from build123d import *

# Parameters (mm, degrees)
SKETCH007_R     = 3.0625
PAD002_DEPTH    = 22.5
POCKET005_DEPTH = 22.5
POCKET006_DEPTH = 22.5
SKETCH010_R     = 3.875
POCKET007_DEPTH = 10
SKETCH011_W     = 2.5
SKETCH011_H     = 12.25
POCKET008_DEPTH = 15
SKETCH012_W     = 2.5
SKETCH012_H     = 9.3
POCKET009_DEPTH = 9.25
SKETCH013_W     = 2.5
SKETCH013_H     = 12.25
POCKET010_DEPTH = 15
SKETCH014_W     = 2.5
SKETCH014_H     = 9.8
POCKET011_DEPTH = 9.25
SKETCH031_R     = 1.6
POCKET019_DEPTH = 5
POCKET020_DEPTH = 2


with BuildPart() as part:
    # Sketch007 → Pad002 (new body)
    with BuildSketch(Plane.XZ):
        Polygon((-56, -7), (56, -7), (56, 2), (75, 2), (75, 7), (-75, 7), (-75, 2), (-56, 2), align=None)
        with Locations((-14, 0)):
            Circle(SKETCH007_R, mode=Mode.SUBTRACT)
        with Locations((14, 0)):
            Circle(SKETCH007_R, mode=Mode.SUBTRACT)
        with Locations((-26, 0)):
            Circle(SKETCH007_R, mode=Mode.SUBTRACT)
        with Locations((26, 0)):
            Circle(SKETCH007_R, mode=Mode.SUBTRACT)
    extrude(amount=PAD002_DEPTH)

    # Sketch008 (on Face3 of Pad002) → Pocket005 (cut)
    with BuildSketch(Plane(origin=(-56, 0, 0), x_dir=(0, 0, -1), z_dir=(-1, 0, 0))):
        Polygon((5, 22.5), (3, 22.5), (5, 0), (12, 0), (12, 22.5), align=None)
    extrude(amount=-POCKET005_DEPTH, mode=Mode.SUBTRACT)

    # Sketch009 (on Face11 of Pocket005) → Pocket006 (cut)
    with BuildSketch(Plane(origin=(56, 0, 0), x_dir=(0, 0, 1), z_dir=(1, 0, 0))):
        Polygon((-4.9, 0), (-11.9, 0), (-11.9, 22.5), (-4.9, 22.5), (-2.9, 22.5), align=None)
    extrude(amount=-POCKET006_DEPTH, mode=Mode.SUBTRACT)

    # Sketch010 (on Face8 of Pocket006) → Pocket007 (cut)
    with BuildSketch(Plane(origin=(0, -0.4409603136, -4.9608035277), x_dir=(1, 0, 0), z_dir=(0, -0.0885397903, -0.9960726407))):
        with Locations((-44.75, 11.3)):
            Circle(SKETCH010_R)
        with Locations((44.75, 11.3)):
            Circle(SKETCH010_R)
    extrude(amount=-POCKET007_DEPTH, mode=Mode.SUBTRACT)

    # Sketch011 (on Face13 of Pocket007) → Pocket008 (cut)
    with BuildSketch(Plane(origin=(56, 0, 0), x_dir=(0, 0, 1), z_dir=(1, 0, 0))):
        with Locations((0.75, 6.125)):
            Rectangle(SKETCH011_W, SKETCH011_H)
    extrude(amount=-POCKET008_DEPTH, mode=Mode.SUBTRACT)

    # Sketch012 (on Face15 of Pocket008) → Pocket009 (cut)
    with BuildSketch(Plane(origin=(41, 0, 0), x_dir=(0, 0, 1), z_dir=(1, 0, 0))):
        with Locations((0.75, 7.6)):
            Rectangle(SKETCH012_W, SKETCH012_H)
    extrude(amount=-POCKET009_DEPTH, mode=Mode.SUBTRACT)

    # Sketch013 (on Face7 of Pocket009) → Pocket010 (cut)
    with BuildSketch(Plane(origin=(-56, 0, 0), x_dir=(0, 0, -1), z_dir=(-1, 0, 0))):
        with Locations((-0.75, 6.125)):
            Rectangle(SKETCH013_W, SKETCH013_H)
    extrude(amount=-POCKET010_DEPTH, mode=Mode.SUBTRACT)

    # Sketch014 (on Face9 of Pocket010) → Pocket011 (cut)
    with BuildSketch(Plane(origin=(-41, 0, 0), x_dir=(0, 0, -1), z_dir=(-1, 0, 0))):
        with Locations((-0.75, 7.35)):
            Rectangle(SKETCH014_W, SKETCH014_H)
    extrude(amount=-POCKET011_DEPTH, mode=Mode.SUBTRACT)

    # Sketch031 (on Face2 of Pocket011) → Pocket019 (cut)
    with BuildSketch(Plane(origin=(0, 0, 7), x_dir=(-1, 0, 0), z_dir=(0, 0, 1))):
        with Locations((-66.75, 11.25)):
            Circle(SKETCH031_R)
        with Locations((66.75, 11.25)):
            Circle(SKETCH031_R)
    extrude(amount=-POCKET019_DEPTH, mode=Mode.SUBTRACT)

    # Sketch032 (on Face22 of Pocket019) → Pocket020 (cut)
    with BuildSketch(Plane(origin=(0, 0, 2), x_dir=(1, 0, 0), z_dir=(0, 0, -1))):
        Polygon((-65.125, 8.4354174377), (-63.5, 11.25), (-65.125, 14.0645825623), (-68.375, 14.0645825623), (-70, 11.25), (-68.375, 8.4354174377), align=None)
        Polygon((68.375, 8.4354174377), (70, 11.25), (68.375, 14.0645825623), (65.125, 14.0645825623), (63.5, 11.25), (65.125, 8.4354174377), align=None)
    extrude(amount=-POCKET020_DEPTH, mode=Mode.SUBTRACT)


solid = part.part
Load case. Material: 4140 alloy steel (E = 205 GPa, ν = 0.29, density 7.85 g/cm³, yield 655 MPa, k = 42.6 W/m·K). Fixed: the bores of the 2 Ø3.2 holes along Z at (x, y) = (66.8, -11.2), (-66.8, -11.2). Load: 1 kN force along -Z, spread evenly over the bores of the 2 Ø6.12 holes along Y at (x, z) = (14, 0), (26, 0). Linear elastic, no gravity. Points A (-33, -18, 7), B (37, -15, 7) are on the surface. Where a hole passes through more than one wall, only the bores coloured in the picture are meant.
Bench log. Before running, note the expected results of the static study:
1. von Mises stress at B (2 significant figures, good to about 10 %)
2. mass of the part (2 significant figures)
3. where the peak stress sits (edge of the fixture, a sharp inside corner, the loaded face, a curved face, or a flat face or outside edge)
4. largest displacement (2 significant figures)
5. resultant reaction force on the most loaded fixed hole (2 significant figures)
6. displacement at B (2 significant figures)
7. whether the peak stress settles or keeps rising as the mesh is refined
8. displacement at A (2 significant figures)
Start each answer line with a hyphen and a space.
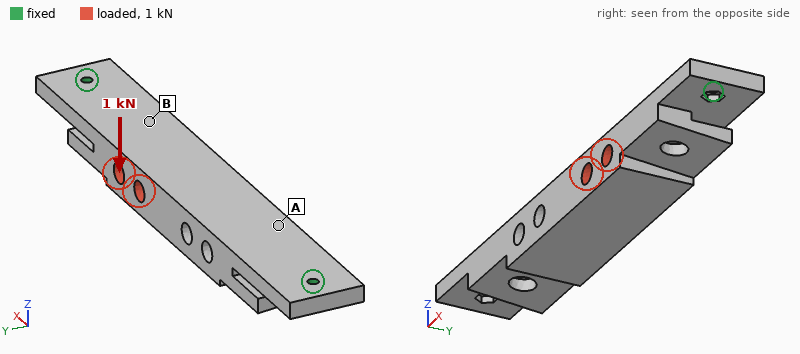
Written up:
- 28 MPa
- 250 g
- edge of the fixture
- 41 µm
- 1.4 kN
- 30 µm
- keeps rising
- 21 µm
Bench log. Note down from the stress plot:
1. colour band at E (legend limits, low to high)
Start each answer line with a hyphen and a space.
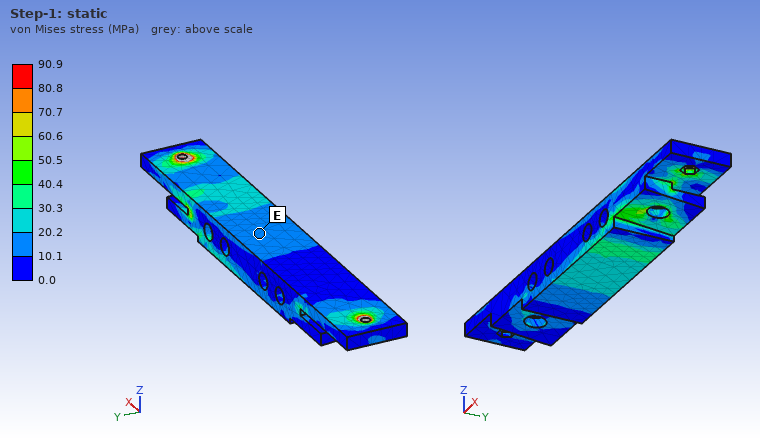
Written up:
- 10.1 to 20.2 MPa
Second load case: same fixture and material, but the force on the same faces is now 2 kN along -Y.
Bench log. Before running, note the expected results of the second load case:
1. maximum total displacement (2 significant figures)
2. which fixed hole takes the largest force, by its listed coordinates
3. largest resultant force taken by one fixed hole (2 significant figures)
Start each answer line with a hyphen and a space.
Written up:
- 73 µm
- (66.8, -11.2)
- 1.3 kN
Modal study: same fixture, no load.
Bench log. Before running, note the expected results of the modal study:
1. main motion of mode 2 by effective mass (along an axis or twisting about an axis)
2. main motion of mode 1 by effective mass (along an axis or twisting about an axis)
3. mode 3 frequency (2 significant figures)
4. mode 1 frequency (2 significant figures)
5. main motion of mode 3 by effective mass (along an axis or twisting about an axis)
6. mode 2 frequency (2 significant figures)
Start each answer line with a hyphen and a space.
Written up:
- along Y
- along Z
- 3700 Hz
- 2000 Hz
- along Y
- 2200 Hz
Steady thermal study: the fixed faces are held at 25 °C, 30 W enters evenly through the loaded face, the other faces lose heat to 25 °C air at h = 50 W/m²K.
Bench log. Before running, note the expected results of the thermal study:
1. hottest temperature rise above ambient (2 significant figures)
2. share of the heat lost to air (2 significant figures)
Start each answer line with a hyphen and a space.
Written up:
- 66 K
- 68 %
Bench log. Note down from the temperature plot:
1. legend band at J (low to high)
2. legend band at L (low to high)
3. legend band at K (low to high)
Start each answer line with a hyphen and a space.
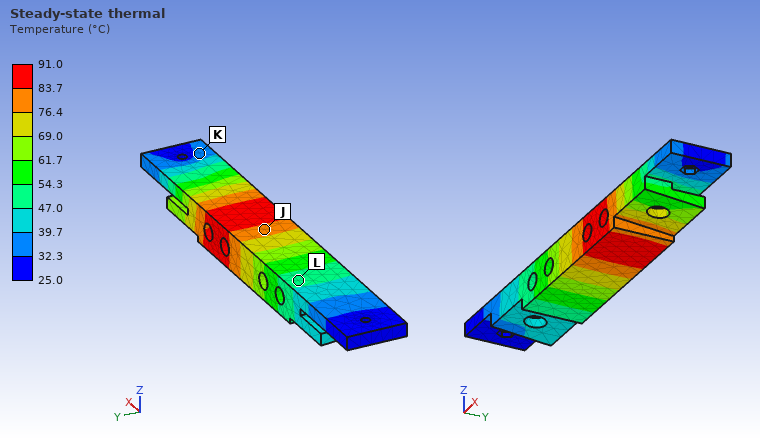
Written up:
- 76.4 to 83.7 °C
- 47.0 to 54.3 °C
- 32.3 to 39.7 °C
